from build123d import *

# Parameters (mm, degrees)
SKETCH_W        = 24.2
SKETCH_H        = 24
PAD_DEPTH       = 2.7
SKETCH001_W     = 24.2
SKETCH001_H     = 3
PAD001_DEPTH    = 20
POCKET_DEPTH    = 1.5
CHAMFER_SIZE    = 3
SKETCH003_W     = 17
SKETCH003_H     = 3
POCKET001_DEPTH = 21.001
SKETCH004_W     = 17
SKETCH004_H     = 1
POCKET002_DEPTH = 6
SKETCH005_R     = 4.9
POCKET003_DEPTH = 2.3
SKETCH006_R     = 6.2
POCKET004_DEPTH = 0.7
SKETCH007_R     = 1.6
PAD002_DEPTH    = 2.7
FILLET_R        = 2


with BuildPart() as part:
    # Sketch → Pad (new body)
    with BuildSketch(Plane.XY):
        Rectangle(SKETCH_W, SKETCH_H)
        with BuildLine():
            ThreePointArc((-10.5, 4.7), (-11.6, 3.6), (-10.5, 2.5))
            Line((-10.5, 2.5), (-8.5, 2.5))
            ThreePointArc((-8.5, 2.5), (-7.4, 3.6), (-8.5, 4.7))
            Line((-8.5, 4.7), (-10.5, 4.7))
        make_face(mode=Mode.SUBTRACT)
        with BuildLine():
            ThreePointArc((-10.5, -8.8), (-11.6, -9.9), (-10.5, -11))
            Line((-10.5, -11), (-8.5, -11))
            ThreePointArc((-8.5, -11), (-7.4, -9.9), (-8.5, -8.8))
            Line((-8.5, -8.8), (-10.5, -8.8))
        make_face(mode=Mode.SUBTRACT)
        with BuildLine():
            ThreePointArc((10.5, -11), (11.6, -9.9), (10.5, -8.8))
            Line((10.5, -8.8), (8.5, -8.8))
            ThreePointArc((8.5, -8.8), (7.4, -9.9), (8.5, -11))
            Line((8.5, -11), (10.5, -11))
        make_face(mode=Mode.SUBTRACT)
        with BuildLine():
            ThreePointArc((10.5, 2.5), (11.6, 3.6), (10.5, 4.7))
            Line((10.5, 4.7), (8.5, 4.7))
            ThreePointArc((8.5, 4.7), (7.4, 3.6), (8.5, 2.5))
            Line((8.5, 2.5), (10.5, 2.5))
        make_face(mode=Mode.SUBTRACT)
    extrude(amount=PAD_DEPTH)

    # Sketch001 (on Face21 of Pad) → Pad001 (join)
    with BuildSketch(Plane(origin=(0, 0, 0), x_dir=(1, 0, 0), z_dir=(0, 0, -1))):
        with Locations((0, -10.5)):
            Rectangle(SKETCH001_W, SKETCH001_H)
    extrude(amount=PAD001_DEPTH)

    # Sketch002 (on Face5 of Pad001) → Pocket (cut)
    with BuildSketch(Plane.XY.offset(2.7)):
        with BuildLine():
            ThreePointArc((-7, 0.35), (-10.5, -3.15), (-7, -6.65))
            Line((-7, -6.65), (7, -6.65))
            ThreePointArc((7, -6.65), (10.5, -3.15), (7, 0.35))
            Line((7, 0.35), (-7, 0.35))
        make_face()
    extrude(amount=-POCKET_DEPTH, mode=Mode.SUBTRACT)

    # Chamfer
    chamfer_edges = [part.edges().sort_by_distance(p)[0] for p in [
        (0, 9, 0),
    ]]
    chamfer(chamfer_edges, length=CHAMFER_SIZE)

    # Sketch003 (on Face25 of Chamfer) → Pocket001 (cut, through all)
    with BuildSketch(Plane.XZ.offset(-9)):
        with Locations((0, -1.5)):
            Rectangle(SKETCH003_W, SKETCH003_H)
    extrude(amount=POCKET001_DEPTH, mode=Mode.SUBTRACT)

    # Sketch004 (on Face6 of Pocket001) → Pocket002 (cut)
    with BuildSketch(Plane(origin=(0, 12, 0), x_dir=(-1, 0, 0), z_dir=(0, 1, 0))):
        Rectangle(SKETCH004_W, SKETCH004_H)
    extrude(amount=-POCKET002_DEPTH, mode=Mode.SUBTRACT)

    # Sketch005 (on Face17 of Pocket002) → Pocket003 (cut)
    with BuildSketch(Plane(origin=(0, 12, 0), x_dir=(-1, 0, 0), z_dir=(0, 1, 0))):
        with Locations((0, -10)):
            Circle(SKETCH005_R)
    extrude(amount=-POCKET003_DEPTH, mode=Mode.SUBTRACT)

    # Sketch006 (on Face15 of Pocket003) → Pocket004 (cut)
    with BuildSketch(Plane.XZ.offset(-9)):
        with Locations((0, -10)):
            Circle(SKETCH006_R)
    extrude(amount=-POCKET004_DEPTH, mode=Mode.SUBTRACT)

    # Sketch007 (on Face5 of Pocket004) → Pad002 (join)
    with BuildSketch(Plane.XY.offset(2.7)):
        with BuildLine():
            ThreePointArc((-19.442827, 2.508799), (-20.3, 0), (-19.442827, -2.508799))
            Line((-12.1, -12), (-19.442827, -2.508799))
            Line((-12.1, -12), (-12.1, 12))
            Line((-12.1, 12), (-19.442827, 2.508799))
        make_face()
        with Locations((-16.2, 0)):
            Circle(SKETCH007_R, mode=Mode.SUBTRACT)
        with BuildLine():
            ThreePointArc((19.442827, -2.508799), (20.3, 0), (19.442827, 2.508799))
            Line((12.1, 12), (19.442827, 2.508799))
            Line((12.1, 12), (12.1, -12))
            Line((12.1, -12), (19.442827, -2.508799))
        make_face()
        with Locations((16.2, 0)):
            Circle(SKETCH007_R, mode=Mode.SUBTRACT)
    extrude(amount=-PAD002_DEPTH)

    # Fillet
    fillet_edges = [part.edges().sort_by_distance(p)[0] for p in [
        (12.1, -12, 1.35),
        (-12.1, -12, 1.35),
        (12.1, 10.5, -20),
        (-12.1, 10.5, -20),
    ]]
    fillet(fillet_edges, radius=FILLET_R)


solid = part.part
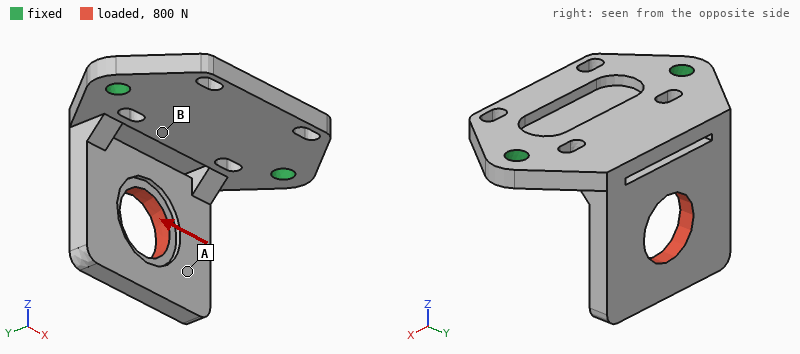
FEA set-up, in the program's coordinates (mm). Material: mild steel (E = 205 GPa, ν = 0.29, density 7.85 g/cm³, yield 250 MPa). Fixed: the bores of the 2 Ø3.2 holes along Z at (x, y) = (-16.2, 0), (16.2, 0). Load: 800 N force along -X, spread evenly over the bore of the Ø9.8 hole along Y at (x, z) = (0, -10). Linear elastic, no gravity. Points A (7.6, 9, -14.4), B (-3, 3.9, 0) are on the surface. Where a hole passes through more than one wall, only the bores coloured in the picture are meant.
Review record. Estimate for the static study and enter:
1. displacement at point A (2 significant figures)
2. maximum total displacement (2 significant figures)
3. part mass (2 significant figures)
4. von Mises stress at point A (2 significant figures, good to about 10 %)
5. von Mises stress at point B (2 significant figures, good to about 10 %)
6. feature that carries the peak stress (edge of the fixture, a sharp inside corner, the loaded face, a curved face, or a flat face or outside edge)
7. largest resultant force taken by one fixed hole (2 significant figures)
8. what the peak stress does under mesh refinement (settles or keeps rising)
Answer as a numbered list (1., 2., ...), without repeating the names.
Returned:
1. 34 µm
2. 46 µm
3. 23 g
4. 21 MPa
5. 51 MPa
6. edge of the fixture
7. 570 N
8. keeps rising
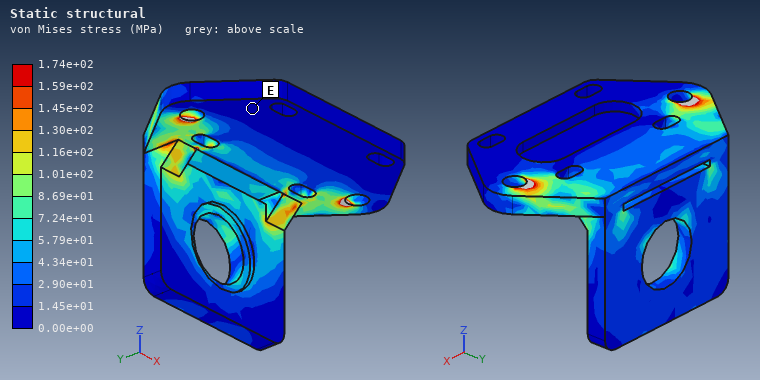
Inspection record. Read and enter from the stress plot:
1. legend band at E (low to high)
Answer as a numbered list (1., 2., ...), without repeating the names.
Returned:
1. 0.00e+00 to 1.45e+01 MPa
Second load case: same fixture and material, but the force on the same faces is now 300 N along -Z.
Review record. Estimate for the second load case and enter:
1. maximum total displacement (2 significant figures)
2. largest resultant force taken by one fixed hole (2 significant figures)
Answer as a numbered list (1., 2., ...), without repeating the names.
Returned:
1. 65 µm
2. 160 N
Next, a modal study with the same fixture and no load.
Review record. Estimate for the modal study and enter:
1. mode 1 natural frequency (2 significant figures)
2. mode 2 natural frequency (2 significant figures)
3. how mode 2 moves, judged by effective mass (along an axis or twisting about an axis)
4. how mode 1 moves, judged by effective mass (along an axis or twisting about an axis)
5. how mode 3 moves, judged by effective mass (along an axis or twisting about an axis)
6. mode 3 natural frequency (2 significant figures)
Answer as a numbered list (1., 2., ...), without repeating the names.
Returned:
1. 2700 Hz
2. 6900 Hz
3. along X
4. along Y
5. along Z
6. 8300 Hz
